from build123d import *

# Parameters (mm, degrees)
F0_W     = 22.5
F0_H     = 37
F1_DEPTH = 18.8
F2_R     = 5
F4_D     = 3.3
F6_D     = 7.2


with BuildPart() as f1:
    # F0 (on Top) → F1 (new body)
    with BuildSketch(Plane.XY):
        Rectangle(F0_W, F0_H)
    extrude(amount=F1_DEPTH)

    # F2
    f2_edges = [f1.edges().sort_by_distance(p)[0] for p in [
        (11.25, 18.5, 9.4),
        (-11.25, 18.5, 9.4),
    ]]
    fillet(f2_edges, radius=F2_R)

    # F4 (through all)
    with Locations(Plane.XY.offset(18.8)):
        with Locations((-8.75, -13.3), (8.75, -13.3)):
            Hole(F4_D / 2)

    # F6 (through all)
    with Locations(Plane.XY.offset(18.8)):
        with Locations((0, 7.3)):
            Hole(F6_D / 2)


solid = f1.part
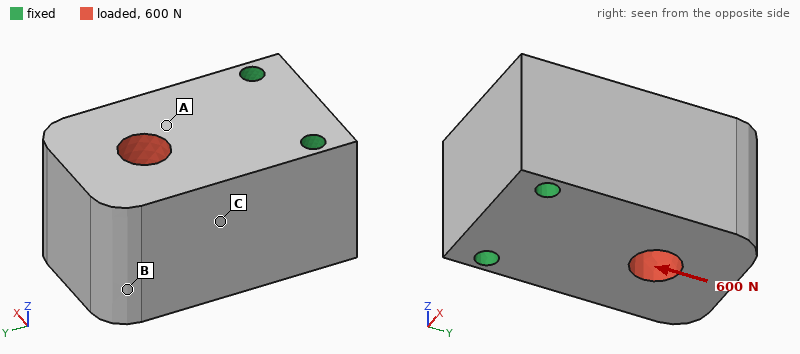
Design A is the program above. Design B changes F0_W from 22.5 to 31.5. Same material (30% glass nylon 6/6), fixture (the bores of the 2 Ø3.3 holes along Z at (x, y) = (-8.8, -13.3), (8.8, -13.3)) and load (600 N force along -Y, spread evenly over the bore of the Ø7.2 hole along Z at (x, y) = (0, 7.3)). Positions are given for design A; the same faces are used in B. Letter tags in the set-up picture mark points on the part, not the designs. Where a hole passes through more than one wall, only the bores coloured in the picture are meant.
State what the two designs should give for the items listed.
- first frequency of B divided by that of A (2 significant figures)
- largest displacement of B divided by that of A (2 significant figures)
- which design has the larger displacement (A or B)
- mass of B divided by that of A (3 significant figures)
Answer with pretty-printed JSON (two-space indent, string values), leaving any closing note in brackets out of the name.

{
  "first frequency of B divided by that of A": "0.96",
  "largest displacement of B divided by that of A": "0.89",
  "which design has the larger displacement": "A",
  "mass of B divided by that of A": "1.44"
}
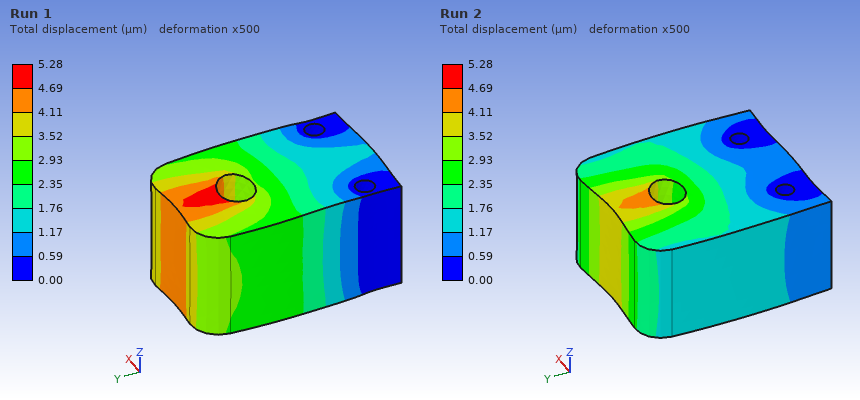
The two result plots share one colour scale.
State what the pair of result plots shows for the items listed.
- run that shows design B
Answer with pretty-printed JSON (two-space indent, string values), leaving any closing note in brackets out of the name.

{
  "run that shows design B": "Run 2"
}
